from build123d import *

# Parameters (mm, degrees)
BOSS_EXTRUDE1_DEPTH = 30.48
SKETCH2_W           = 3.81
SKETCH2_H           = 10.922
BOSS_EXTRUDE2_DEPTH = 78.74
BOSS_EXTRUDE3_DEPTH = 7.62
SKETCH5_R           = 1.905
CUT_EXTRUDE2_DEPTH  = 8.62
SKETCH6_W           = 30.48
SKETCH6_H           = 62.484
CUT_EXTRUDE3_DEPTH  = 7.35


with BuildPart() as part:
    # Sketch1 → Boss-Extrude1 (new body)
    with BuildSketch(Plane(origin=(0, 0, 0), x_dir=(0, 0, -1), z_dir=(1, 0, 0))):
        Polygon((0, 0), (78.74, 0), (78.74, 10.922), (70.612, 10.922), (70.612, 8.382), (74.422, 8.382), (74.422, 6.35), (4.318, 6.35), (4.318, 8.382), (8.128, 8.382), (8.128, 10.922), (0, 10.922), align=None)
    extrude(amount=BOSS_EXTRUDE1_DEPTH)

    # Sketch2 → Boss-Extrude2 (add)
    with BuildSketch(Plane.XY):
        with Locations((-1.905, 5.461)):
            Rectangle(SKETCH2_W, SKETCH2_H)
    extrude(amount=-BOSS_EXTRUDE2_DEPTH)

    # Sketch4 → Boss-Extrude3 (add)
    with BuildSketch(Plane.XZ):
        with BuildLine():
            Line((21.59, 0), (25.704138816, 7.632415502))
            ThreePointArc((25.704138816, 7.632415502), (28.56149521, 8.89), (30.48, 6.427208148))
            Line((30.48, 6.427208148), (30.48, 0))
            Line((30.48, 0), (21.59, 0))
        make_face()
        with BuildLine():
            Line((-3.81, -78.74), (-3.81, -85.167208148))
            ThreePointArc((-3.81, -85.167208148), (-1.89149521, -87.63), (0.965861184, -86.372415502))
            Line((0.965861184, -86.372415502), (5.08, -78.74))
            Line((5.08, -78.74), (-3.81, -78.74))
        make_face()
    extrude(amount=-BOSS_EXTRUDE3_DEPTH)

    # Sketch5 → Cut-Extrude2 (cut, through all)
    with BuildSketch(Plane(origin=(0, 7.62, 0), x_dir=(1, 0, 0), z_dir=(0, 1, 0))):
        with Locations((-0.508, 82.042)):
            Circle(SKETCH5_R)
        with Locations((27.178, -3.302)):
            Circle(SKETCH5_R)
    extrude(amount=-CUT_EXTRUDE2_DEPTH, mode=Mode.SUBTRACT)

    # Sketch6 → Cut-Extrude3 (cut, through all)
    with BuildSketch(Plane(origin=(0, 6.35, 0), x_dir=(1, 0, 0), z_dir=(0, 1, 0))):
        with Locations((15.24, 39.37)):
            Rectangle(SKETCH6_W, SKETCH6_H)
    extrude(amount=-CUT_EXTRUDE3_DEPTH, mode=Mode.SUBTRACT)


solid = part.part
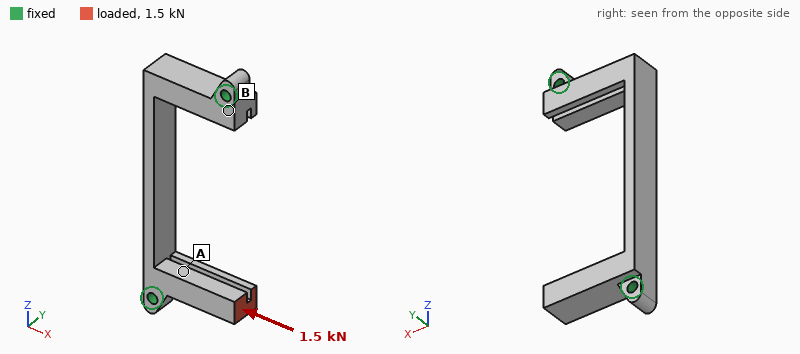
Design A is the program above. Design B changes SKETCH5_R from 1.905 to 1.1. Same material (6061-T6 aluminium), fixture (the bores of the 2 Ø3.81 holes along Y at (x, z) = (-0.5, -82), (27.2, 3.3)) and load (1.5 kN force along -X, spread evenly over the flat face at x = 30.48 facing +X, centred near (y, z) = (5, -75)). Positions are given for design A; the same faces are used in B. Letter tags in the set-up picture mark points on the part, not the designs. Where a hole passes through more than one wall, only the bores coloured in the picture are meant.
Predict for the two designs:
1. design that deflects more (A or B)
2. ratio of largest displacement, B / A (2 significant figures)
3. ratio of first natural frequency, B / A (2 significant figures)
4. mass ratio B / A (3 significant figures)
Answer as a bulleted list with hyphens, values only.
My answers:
- B
- 1.8
- 0.88
- 1.01
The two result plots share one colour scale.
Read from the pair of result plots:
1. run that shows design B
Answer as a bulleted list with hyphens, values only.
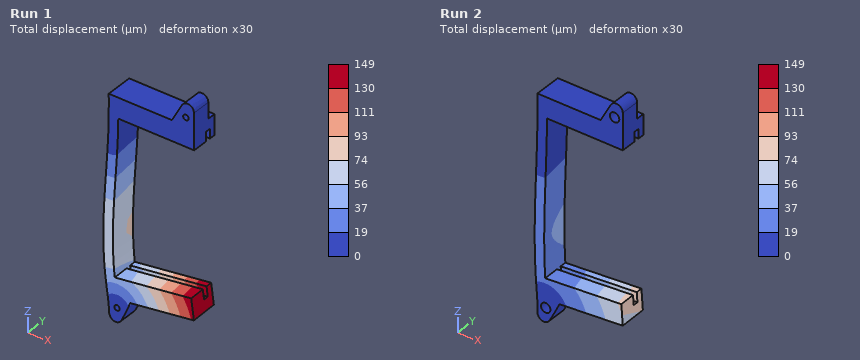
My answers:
- Run 1
